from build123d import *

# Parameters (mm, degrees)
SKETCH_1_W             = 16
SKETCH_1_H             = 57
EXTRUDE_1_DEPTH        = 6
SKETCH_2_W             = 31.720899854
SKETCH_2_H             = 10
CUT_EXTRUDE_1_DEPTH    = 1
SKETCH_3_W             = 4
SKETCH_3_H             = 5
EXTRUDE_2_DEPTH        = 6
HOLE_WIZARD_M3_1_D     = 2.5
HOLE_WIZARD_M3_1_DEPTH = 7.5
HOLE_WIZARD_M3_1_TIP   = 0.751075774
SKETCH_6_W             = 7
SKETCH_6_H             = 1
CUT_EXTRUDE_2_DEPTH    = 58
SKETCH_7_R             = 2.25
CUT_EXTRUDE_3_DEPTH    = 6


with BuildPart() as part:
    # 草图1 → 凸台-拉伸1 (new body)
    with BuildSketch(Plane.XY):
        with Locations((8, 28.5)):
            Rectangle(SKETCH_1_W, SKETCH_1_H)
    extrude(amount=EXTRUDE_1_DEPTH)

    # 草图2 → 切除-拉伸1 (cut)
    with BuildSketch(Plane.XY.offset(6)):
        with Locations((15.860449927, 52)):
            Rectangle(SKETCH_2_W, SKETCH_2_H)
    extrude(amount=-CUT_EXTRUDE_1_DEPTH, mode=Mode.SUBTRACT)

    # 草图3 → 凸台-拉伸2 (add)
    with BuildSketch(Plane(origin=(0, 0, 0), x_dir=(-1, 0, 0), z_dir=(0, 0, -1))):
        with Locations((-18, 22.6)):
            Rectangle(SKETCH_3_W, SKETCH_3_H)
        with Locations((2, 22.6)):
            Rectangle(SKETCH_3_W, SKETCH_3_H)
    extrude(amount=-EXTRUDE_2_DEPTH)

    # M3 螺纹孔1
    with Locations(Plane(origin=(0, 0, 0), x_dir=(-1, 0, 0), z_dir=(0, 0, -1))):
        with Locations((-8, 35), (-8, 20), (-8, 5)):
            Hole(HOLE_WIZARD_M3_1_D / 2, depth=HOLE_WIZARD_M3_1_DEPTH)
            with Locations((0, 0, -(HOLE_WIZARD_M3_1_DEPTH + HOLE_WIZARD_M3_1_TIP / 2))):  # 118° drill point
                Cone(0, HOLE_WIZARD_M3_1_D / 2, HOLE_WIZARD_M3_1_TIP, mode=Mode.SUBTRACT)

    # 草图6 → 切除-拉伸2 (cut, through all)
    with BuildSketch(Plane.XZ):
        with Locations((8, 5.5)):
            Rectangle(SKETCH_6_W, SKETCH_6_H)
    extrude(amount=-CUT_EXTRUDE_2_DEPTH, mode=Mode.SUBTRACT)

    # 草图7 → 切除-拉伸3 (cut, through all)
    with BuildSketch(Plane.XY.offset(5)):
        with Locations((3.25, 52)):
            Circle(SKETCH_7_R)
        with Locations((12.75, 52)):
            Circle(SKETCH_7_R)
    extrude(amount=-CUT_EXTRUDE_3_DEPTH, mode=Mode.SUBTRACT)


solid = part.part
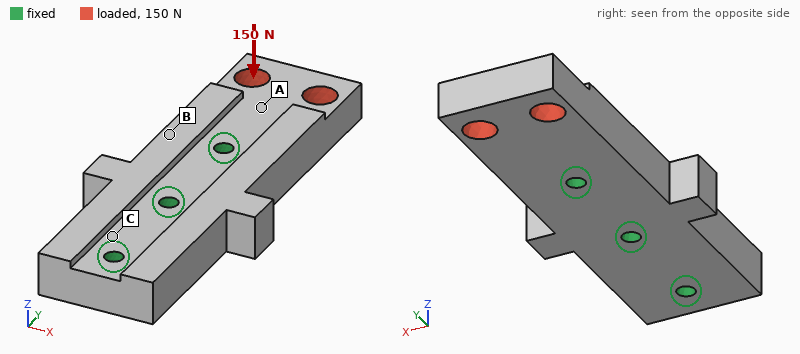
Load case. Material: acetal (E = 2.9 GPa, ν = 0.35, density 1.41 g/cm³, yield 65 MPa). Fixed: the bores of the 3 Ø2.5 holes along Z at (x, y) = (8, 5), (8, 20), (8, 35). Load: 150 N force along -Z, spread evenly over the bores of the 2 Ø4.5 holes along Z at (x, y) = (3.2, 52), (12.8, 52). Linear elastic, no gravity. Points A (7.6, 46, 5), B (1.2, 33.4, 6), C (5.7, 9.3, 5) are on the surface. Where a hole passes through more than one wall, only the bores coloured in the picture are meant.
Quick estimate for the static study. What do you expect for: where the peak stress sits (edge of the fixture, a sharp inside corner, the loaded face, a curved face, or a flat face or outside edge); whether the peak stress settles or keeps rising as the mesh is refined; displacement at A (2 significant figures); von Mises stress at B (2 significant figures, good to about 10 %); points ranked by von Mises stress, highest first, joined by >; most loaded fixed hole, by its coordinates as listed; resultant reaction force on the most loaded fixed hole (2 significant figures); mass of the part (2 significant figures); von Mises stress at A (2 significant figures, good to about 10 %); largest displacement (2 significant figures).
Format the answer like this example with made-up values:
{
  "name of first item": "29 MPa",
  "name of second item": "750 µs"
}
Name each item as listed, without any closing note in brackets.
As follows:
{
  "where the peak stress sits": "edge of the fixture",
  "whether the peak stress settles or keeps rising as the mesh is refined": "keeps rising",
  "displacement at A": "0.27 mm",
  "von Mises stress at B": "16 MPa",
  "points ranked by von Mises stress, highest first, joined by >": "B > A > C",
  "most loaded fixed hole, by its coordinates as listed": "(8, 35)",
  "resultant reaction force on the most loaded fixed hole": "230 N",
  "mass of the part": "7.0 g",
  "von Mises stress at A": "9.6 MPa",
  "largest displacement": "0.70 mm"
}
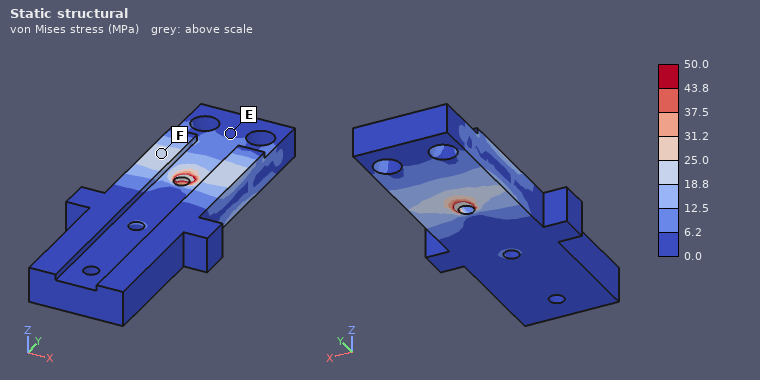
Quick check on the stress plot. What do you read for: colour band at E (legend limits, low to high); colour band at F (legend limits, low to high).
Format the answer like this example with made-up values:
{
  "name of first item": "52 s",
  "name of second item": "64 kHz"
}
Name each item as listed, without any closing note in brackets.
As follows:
{
  "colour band at E": "0.0 to 6.2 MPa",
  "colour band at F": "18.8 to 25.0 MPa"
}
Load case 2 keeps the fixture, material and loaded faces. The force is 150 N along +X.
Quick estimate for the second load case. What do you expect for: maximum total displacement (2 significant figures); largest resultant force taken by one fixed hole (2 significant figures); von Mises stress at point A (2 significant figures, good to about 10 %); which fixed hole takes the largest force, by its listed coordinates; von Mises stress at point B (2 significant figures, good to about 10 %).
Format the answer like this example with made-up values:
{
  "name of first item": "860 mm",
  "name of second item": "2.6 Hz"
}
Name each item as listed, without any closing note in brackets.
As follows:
{
  "maximum total displacement": "0.20 mm",
  "largest resultant force taken by one fixed hole": "270 N",
  "von Mises stress at point A": "4.6 MPa",
  "which fixed hole takes the largest force, by its listed coordinates": "(8, 35)",
  "von Mises stress at point B": "7.2 MPa"
}
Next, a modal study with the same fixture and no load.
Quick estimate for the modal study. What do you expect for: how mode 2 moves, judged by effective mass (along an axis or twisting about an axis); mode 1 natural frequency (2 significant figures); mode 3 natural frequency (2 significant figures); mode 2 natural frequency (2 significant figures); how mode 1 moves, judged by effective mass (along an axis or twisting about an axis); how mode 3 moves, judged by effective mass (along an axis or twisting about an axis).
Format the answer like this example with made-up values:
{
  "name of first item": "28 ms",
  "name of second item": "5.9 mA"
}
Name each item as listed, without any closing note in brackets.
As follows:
{
  "how mode 2 moves, judged by effective mass": "along X",
  "mode 1 natural frequency": "2600 Hz",
  "mode 3 natural frequency": "5400 Hz",
  "mode 2 natural frequency": "4500 Hz",
  "how mode 1 moves, judged by effective mass": "along Z",
  "how mode 3 moves, judged by effective mass": "twisting about Y"
}
